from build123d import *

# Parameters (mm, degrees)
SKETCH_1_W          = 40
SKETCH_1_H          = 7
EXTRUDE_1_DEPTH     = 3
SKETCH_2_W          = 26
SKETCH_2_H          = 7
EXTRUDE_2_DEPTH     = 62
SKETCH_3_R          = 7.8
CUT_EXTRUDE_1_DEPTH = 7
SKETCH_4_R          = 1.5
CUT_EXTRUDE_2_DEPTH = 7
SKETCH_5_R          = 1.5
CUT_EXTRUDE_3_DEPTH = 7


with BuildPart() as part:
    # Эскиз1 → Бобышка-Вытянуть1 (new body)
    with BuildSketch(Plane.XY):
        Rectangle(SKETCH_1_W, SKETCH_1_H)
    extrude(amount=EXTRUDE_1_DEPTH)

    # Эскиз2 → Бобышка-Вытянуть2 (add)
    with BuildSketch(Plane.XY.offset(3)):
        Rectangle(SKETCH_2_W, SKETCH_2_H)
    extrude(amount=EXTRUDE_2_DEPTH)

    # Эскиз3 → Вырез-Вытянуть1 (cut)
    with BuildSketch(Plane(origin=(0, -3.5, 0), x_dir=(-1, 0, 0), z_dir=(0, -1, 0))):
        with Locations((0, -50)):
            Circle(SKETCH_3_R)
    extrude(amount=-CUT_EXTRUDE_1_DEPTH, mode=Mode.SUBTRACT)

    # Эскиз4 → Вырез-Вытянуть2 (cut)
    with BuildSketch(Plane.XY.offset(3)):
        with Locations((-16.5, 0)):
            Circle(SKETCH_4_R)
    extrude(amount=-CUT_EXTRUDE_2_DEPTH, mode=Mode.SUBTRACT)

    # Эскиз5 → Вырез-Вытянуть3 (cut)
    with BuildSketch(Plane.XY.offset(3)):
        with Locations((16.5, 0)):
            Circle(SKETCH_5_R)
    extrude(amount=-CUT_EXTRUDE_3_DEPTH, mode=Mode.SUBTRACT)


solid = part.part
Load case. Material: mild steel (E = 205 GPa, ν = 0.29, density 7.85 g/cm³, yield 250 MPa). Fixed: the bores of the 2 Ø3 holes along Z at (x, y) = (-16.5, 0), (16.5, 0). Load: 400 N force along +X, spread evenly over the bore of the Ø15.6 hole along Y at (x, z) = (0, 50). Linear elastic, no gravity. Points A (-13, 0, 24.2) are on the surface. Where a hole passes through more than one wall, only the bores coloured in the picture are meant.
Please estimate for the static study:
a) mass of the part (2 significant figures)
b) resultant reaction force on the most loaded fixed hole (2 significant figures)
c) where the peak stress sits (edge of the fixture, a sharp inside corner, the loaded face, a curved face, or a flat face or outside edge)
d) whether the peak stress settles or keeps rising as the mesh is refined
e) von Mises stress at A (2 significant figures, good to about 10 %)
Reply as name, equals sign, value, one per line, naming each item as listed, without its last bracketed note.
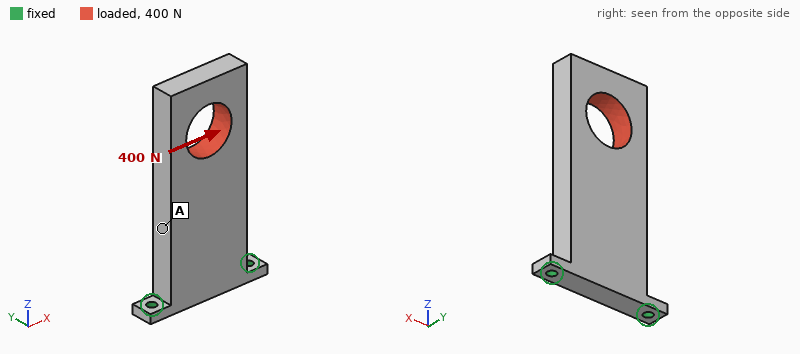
mass of the part = 84 g
resultant reaction force on the most loaded fixed hole = 730 N
where the peak stress sits = edge of the fixture
whether the peak stress settles or keeps rising as the mesh is refined = keeps rising
von Mises stress at A = 13 MPa
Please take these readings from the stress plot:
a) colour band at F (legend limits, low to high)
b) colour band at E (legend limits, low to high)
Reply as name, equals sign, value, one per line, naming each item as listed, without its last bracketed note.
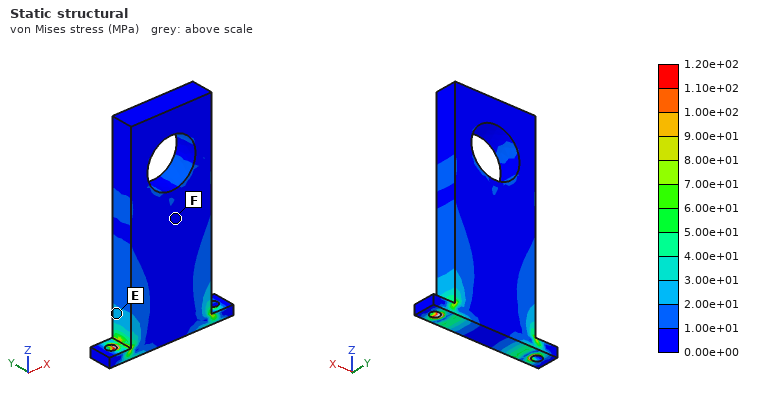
colour band at F = 0.00e+00 to 1.00e+01 MPa
colour band at E = 2.00e+01 to 3.00e+01 MPa
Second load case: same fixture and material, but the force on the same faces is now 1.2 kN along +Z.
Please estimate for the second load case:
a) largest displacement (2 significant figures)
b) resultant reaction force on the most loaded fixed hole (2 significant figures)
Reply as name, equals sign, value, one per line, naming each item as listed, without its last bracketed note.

largest displacement = 6.0 µm
resultant reaction force on the most loaded fixed hole = 670 N
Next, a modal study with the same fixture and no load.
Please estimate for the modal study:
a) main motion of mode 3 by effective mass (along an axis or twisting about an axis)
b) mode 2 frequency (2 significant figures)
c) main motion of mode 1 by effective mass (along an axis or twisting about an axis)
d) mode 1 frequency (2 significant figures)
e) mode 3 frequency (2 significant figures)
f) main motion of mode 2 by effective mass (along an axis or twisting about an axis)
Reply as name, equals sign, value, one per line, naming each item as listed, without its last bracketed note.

main motion of mode 3 by effective mass = twisting about Z
mode 2 frequency = 3400 Hz
main motion of mode 1 by effective mass = along Y
mode 1 frequency = 710 Hz
mode 3 frequency = 5800 Hz
main motion of mode 2 by effective mass = along X
